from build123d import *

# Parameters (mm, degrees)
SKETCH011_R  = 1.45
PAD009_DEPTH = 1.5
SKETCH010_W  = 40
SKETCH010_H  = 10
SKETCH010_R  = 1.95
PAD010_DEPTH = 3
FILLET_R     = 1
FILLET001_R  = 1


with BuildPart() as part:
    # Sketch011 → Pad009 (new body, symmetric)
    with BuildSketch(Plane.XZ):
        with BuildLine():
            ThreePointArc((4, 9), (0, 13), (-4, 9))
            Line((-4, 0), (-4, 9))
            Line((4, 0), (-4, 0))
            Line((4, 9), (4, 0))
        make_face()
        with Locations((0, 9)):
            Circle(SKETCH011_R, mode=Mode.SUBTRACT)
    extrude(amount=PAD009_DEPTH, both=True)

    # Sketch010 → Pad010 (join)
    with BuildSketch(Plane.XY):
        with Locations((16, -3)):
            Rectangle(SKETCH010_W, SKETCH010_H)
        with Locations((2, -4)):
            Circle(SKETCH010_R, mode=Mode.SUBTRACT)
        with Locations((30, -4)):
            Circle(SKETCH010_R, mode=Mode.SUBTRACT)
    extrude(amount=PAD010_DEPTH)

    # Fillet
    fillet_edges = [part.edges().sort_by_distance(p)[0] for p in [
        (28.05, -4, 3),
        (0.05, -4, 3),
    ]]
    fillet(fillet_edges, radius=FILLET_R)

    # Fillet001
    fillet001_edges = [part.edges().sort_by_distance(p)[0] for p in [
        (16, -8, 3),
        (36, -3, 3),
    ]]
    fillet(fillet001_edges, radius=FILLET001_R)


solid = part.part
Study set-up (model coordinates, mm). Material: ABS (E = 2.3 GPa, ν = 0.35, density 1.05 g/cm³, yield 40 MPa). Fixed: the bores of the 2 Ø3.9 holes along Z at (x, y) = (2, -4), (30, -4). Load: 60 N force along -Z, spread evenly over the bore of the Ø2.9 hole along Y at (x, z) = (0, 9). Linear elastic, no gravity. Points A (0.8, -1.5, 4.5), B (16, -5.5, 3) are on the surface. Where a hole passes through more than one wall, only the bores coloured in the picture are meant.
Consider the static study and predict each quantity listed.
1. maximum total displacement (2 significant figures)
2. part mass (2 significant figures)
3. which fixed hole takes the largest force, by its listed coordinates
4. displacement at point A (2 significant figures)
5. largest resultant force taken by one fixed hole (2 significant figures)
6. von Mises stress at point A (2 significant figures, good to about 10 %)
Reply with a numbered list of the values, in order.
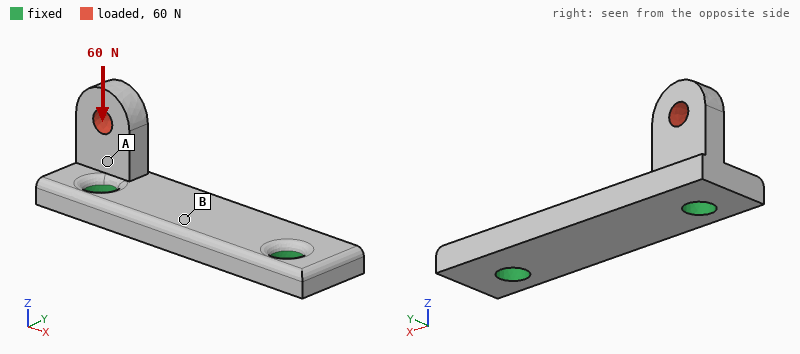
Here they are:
1. 0.14 mm
2. 1.4 g
3. (2, -4)
4. 0.038 mm
5. 61 N
6. 3.4 MPa
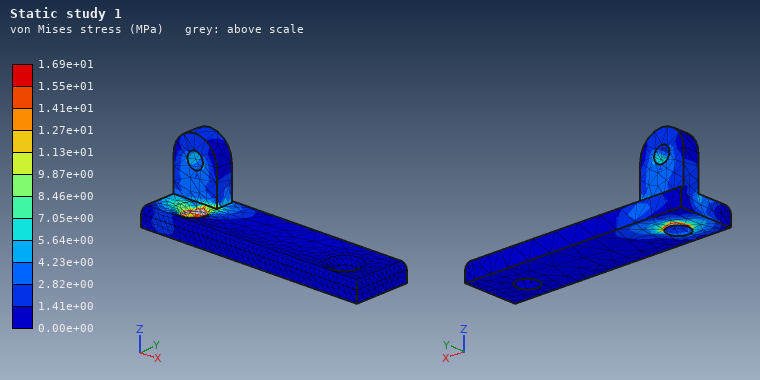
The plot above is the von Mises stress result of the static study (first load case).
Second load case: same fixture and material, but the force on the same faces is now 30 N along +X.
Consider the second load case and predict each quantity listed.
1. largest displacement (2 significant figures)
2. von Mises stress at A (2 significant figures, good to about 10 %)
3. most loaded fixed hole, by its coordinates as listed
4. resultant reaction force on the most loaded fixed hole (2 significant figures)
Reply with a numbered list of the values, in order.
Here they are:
1. 0.15 mm
2. 5.8 MPa
3. (2, -4)
4. 23 N
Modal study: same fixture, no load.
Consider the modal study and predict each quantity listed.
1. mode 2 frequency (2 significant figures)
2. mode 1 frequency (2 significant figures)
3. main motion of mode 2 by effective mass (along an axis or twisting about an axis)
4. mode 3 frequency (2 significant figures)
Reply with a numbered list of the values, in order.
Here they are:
1. 5400 Hz
2. 4500 Hz
3. along Z
4. 6800 Hz
